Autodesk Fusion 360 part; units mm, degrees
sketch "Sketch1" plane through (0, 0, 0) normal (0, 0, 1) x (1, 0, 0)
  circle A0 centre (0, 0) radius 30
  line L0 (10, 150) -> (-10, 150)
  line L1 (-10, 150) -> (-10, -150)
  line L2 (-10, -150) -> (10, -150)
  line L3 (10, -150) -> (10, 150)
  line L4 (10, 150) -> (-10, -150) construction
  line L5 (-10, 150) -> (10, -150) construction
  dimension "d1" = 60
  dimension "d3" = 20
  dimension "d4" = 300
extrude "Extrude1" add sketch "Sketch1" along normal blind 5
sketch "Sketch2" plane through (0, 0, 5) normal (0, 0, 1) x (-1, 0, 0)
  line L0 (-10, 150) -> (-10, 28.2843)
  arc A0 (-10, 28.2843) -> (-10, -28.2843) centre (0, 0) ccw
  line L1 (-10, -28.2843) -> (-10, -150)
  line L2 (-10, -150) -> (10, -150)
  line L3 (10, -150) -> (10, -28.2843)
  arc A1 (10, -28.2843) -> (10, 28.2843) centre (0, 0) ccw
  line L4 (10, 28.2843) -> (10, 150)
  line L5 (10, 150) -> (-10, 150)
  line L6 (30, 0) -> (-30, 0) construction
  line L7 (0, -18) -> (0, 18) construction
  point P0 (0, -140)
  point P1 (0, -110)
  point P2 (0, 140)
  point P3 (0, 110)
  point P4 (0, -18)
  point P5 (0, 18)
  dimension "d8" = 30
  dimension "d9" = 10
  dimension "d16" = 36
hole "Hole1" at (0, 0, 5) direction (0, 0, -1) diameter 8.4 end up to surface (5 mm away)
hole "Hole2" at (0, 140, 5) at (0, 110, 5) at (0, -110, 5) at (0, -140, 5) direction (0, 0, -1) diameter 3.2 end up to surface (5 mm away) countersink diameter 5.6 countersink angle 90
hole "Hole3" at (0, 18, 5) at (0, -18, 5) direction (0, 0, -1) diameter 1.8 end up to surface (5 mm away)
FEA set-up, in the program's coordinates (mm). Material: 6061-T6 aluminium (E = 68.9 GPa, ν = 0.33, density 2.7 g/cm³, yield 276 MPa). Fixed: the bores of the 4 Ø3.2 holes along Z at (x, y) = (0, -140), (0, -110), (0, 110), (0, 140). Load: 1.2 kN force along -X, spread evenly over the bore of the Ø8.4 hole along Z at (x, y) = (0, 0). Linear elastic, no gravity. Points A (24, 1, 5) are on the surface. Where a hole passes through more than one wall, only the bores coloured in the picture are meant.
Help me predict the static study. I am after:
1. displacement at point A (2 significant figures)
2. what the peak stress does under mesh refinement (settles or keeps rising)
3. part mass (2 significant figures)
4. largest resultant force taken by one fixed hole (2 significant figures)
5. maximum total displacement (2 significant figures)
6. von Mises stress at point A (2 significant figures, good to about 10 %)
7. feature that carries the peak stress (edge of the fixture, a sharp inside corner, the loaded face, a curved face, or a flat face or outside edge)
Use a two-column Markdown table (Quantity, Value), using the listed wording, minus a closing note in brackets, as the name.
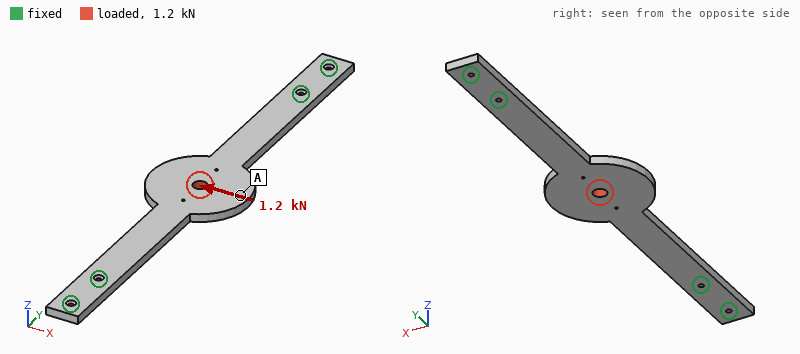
| Quantity | Value |
|---|---|
| displacement at point A | 0.23 mm |
| what the peak stress does under mesh refinement | keeps rising |
| part mass | 100 g |
| largest resultant force taken by one fixed hole | 1.3 kN |
| maximum total displacement | 0.23 mm |
| von Mises stress at point A | 10 MPa |
| feature that carries the peak stress | edge of the fixture |
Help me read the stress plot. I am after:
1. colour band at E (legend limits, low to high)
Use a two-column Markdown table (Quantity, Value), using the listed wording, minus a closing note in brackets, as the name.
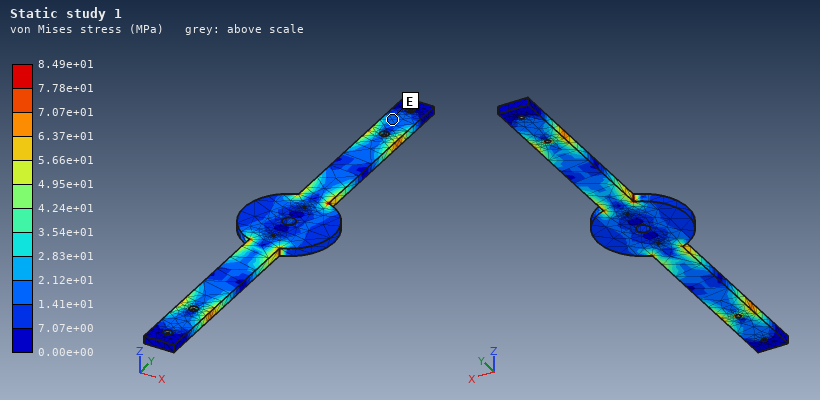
| Quantity | Value |
|---|---|
| colour band at E | 1.41e+01 to 2.12e+01 MPa |
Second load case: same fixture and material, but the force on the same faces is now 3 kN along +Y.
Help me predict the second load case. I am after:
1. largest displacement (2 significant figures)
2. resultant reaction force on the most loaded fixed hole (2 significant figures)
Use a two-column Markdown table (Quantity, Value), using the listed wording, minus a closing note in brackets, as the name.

| Quantity | Value |
|---|---|
| largest displacement | 25 µm |
| resultant reaction force on the most loaded fixed hole | 1.3 kN |
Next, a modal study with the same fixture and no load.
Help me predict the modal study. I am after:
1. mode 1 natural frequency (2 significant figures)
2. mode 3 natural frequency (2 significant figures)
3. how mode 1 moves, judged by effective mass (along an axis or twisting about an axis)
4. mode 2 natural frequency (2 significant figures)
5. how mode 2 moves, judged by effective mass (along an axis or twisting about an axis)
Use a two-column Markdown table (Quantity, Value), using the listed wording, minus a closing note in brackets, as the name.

| Quantity | Value |
|---|---|
| mode 1 natural frequency | 420 Hz |
| mode 3 natural frequency | 1400 Hz |
| how mode 1 moves, judged by effective mass | along Z |
| mode 2 natural frequency | 1100 Hz |
| how mode 2 moves, judged by effective mass | twisting about Y |
